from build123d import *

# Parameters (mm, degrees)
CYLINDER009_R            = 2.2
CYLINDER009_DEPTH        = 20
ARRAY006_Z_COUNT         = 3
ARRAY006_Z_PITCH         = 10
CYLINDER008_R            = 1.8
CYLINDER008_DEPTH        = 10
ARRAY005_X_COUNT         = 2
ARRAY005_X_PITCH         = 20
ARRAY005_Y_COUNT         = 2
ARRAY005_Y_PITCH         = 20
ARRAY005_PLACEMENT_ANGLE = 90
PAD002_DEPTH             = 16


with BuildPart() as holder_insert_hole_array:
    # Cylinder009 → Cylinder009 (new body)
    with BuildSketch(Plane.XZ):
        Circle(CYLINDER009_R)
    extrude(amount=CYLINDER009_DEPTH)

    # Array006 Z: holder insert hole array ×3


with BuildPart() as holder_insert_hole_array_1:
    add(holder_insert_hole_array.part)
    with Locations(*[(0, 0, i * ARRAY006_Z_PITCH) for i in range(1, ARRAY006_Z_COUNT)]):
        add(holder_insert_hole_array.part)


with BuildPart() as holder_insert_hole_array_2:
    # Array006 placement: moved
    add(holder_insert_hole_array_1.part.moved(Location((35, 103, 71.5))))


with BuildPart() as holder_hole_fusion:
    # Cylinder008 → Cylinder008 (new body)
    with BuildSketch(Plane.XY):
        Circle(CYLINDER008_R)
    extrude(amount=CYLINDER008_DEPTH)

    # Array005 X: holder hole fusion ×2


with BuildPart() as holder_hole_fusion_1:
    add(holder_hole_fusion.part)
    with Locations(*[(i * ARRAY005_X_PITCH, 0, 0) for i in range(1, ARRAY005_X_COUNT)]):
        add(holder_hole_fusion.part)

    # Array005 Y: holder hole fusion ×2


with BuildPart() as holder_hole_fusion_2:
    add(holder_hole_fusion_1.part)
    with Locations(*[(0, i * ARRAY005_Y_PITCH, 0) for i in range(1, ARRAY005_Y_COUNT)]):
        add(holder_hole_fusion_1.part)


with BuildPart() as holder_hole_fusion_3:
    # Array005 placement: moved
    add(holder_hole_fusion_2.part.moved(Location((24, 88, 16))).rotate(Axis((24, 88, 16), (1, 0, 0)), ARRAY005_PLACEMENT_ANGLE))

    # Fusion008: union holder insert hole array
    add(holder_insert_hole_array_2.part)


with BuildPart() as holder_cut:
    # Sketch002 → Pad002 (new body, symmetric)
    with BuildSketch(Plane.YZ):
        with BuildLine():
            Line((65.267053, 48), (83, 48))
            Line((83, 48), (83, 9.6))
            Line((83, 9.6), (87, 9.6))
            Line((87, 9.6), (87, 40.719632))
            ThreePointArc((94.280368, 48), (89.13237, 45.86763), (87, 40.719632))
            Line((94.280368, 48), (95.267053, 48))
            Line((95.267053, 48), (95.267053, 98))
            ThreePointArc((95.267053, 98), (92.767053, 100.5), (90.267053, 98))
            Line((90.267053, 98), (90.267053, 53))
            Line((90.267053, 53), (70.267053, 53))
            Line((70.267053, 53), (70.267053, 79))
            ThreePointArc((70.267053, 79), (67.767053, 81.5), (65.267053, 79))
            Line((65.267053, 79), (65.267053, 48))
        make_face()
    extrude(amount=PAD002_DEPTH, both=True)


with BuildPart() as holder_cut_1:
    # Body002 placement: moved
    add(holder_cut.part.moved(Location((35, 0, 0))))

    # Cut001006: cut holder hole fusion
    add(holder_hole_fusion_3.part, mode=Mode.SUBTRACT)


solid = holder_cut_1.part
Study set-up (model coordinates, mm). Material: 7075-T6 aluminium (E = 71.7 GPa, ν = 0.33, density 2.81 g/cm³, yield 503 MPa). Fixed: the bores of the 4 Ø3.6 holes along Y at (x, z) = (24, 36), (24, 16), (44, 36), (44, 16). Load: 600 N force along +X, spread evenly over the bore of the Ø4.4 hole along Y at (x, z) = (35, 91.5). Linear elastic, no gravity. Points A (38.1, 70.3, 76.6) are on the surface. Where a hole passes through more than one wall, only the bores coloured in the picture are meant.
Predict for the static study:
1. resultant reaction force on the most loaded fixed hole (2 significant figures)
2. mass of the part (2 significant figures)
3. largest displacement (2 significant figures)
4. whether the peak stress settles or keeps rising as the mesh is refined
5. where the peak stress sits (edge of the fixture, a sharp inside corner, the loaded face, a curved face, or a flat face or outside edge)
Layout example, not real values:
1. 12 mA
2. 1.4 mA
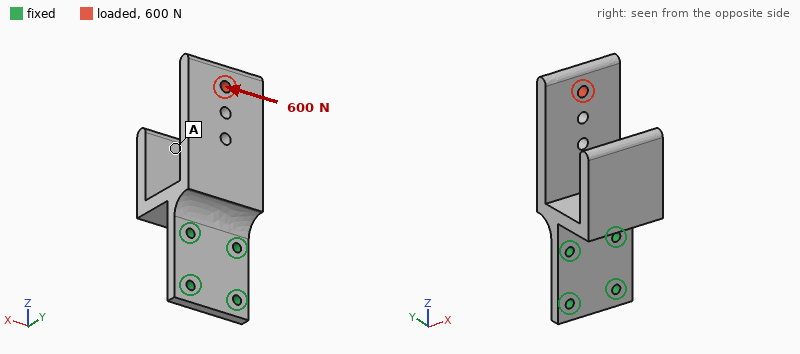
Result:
1. 1.4 kN
2. 61 g
3. 0.10 mm
4. keeps rising
5. edge of the fixture
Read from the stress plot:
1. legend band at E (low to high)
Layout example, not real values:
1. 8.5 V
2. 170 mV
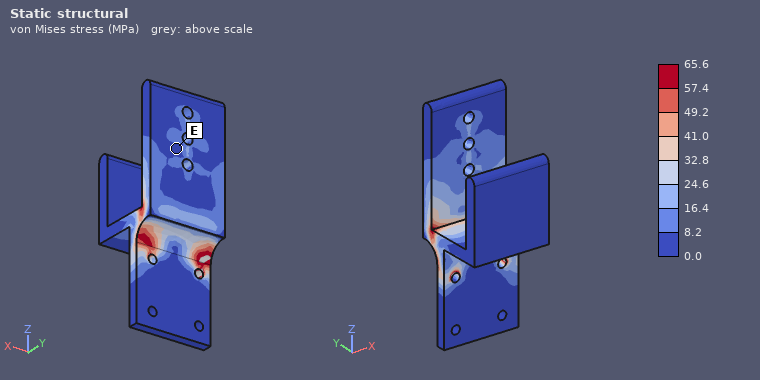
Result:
1. 0.0 to 8.2 MPa
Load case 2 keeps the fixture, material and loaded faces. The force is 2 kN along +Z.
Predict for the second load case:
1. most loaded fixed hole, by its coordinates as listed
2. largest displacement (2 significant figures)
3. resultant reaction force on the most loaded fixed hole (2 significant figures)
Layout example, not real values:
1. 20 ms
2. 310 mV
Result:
1. (44, 36)
2. 0.69 mm
3. 950 N
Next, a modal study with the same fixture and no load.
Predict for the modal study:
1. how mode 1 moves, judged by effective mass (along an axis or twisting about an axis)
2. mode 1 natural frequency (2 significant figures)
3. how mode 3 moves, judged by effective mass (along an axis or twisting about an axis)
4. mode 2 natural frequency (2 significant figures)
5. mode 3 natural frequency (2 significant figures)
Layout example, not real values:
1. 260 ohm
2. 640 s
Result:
1. along Y
2. 780 Hz
3. along X
4. 2000 Hz
5. 3300 Hz
